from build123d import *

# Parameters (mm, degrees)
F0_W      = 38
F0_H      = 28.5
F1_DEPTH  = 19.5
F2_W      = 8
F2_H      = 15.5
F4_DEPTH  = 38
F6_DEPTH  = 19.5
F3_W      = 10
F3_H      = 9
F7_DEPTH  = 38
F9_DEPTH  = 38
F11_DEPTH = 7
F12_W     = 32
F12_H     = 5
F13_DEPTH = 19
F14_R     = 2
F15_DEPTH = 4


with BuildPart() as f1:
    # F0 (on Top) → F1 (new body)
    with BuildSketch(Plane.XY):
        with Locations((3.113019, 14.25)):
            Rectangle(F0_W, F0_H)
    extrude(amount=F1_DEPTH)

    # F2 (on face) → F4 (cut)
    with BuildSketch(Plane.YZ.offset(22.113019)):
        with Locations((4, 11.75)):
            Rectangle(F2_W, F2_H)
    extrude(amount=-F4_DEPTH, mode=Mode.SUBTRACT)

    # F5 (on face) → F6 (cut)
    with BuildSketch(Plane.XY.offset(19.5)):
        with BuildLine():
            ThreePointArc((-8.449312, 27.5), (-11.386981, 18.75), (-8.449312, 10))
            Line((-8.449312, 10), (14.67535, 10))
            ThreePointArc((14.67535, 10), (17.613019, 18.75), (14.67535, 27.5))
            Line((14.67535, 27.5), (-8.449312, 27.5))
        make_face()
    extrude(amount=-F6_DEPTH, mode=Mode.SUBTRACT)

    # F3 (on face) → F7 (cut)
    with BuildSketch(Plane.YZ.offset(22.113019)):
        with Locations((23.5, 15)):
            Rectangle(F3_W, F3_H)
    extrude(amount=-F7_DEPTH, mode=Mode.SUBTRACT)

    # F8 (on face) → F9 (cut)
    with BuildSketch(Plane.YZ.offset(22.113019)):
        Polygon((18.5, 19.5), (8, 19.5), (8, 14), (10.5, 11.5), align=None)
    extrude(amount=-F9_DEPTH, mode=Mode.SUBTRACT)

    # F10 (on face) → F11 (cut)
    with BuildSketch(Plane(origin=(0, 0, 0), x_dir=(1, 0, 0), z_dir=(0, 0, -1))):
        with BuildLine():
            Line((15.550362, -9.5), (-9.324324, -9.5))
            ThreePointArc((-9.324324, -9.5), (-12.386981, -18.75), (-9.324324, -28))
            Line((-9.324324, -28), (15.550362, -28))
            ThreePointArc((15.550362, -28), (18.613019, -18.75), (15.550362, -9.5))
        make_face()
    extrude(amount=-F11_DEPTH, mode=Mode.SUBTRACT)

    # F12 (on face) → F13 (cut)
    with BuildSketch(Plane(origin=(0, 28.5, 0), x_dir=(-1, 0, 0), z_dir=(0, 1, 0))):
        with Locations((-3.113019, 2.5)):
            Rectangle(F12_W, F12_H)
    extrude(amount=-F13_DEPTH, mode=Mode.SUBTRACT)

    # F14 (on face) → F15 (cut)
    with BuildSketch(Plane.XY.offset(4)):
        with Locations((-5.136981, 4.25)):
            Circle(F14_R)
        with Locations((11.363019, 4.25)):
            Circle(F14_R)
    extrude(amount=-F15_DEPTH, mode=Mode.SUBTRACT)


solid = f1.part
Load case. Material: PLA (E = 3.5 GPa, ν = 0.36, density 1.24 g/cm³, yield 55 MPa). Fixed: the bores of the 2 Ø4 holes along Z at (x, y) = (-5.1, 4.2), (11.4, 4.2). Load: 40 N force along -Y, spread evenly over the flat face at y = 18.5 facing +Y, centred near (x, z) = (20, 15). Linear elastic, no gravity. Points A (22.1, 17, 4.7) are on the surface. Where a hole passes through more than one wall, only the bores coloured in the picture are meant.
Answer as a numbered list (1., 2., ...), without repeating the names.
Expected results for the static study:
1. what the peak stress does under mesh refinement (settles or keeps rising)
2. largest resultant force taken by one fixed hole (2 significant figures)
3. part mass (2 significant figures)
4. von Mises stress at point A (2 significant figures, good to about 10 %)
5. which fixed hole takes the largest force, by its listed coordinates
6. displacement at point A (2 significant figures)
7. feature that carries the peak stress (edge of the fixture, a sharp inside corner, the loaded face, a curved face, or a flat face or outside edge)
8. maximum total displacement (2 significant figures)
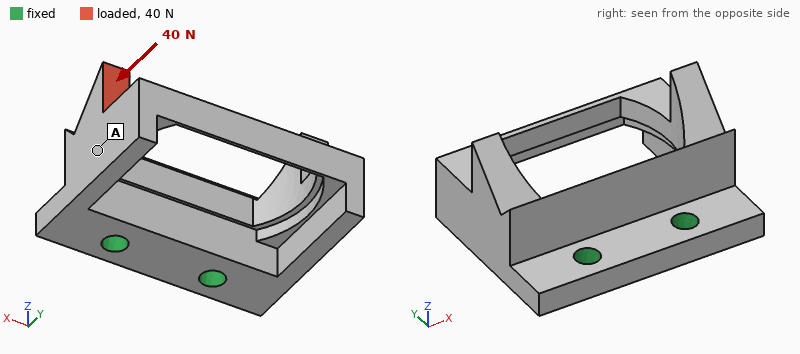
1. keeps rising
2. 46 N
3. 5.1 g
4. 3.6 MPa
5. (11.4, 4.2)
6. 0.25 mm
7. a sharp inside corner
8. 0.56 mm
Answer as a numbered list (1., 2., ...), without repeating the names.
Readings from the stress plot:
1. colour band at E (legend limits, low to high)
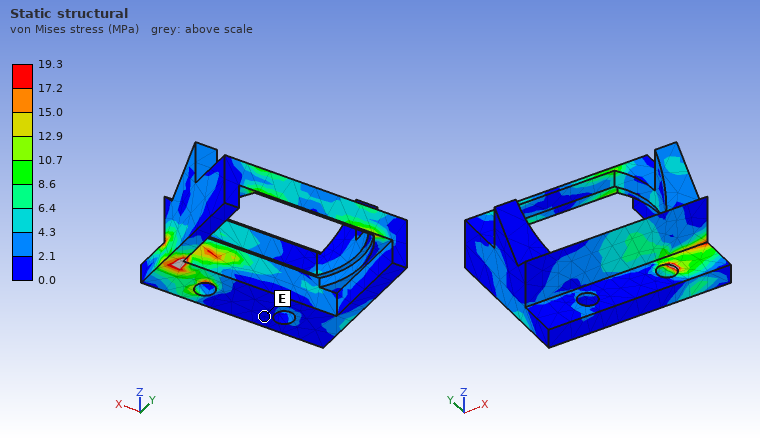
1. 0.0 to 2.1 MPa
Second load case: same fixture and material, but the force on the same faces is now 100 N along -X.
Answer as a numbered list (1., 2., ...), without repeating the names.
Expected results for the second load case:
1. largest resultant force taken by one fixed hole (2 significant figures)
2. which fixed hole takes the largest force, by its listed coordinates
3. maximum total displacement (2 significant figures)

1. 96 N
2. (-5.1, 4.2)
3. 0.57 mm
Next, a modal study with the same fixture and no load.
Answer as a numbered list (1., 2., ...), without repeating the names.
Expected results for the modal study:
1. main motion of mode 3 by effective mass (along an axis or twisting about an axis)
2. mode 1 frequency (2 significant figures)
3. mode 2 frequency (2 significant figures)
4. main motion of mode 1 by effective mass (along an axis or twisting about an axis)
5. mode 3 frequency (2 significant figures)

1. along X
2. 1300 Hz
3. 1400 Hz
4. along Z
5. 1900 Hz
